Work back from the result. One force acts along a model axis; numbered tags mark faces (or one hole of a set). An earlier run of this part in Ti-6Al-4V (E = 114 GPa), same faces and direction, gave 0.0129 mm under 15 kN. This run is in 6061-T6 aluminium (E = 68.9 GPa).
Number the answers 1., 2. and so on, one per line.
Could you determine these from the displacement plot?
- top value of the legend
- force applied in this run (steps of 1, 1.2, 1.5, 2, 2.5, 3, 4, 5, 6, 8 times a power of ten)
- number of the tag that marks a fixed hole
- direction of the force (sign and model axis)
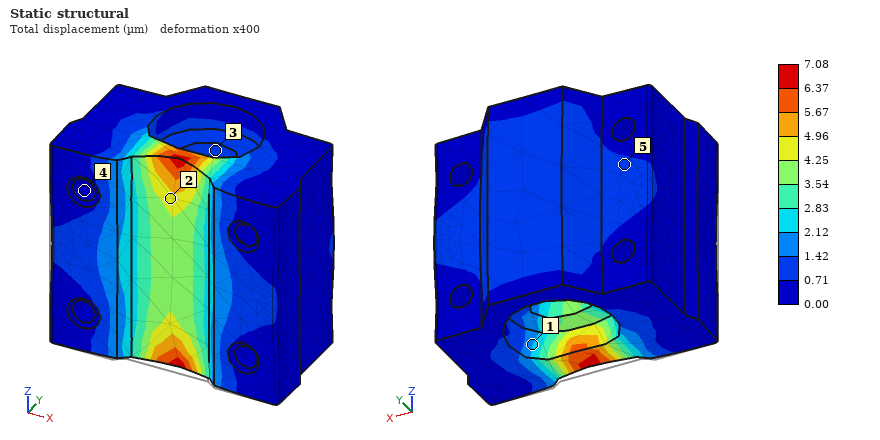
1. 7.08 µm
2. 5 kN
3. 4
4. +Y
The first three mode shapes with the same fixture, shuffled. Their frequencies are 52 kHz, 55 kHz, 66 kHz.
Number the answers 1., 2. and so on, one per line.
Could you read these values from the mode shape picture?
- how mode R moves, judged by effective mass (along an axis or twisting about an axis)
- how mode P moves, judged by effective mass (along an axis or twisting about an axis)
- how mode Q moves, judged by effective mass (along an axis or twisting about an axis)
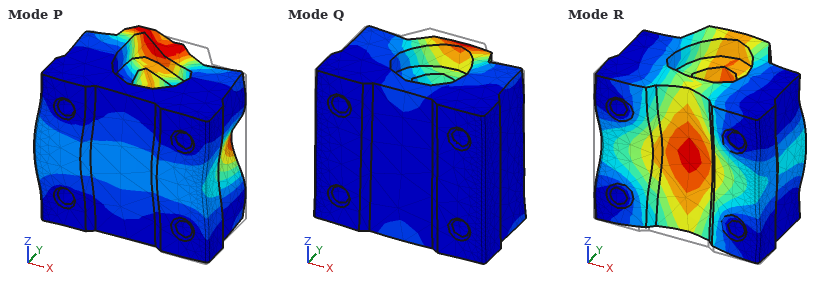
1. along Y
2. along X
3. along Z
